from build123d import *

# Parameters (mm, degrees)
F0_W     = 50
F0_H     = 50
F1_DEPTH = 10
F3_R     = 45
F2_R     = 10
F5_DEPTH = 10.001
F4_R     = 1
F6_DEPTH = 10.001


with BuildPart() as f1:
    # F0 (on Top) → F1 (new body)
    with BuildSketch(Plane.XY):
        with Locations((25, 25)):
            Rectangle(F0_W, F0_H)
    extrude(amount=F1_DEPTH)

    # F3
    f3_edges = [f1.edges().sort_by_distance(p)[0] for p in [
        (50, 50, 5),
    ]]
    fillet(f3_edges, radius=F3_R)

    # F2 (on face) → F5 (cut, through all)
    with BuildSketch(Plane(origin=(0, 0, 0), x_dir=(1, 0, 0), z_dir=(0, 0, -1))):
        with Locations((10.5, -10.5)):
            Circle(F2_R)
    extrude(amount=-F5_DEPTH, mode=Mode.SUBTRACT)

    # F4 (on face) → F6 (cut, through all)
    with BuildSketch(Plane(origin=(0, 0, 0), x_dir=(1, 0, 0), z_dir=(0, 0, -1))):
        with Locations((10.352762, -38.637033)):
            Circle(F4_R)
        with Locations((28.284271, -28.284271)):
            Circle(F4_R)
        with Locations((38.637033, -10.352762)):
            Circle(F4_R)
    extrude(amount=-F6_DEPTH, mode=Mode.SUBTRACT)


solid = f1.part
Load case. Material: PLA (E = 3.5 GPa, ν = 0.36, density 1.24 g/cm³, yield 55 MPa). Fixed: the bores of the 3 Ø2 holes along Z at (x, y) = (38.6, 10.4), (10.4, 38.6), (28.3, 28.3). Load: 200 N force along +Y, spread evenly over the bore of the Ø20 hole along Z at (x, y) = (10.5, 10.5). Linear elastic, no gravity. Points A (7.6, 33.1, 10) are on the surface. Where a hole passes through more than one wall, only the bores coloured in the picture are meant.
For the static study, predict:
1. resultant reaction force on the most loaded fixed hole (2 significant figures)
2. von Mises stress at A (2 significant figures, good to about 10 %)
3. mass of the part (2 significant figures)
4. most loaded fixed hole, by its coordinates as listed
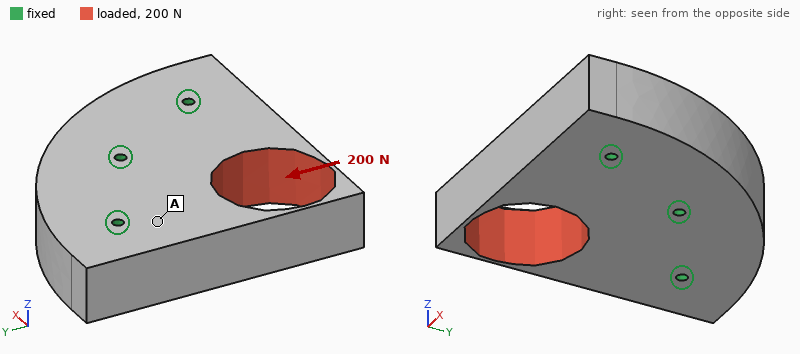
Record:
140 N
1.2 MPa
22 g
(10.4, 38.6)
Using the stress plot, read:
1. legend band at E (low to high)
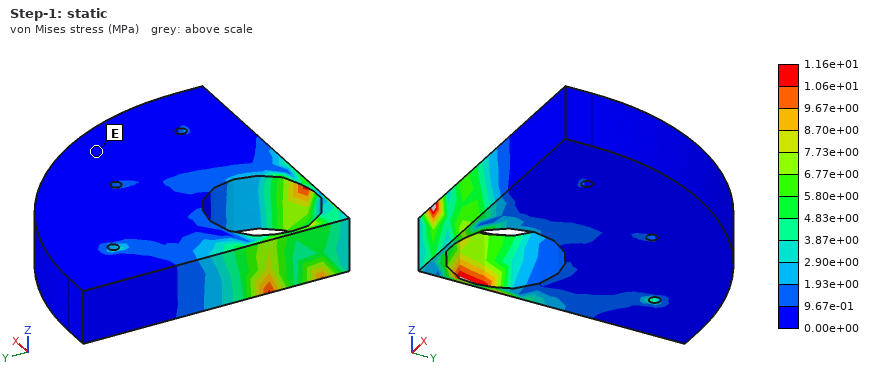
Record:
0.00e+00 to 9.67e-01 MPa
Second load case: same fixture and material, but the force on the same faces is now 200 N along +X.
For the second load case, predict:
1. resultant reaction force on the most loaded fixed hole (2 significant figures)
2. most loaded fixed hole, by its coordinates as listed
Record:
140 N
(38.6, 10.4)
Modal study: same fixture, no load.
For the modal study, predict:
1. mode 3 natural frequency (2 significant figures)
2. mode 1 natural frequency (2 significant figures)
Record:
6700 Hz
3600 Hz
